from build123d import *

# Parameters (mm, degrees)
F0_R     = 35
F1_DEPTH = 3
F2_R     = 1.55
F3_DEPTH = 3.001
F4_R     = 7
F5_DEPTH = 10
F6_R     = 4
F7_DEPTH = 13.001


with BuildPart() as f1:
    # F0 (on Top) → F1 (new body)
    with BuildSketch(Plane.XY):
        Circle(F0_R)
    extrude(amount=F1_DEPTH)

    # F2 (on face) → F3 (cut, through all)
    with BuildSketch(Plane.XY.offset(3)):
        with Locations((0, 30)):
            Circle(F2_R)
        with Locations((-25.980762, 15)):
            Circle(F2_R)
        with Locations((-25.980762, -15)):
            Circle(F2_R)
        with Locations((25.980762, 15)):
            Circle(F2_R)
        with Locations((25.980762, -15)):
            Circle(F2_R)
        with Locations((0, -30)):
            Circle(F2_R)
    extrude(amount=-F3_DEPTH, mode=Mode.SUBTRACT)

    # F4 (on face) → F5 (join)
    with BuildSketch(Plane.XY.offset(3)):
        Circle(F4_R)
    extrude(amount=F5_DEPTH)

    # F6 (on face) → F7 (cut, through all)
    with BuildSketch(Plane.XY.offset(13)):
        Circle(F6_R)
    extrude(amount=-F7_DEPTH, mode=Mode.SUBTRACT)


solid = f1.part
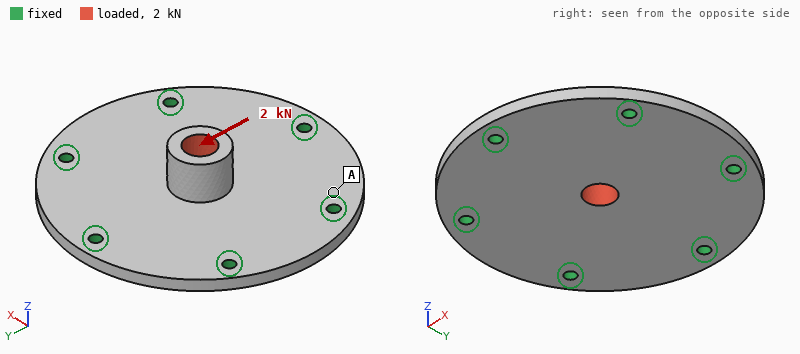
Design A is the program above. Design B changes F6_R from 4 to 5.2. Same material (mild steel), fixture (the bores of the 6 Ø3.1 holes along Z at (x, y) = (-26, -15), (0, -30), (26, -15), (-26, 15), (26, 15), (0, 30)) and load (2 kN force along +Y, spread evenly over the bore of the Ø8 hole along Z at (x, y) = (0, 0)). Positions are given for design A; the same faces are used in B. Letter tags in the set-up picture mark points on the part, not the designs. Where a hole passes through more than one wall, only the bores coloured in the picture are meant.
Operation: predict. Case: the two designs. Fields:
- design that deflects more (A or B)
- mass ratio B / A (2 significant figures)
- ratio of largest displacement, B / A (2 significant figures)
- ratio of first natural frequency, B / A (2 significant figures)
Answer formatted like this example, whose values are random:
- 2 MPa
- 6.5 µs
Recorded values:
- B
- 0.96
- 1.2
- 1.0
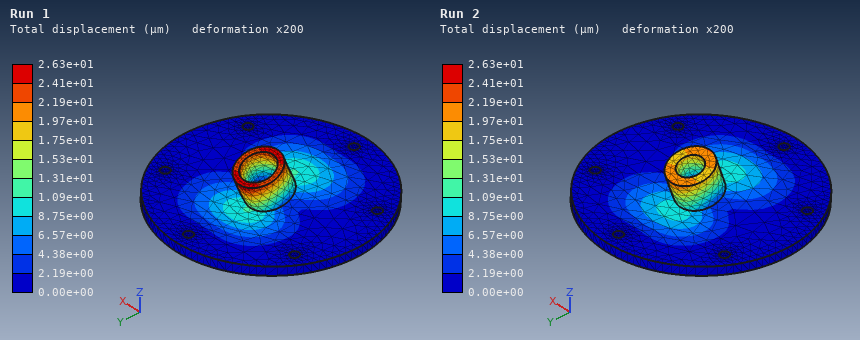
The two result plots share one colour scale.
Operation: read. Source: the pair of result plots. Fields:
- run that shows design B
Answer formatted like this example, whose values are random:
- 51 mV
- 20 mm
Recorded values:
- Run 1
